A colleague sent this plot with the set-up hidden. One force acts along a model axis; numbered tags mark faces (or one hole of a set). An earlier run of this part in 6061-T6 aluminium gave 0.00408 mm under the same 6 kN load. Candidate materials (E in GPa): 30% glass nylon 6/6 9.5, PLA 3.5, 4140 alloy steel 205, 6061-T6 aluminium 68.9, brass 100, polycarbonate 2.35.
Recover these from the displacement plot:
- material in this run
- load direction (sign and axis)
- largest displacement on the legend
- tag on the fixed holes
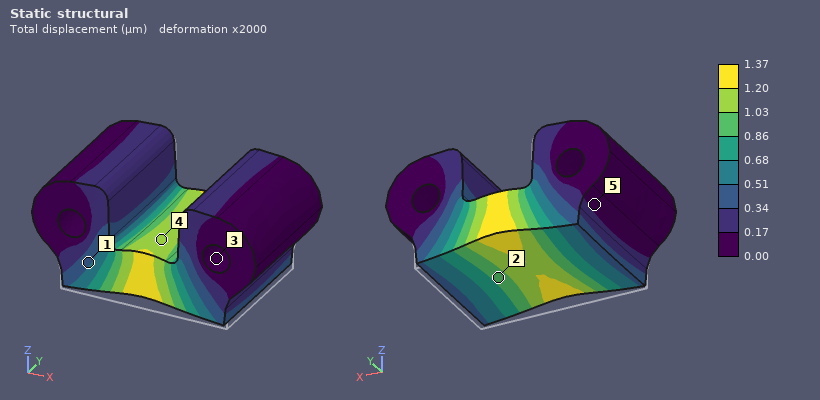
4140 alloy steel
+Z
1.37 µm
3
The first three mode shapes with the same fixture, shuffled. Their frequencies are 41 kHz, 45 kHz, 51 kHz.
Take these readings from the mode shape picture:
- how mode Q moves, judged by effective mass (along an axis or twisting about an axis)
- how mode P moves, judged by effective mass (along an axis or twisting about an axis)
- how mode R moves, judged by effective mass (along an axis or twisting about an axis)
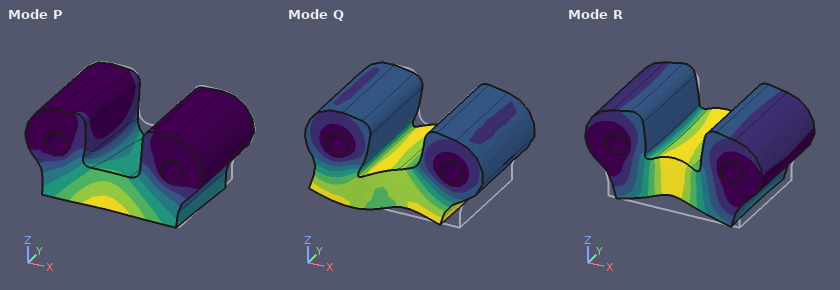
along X
along Y
along Z
